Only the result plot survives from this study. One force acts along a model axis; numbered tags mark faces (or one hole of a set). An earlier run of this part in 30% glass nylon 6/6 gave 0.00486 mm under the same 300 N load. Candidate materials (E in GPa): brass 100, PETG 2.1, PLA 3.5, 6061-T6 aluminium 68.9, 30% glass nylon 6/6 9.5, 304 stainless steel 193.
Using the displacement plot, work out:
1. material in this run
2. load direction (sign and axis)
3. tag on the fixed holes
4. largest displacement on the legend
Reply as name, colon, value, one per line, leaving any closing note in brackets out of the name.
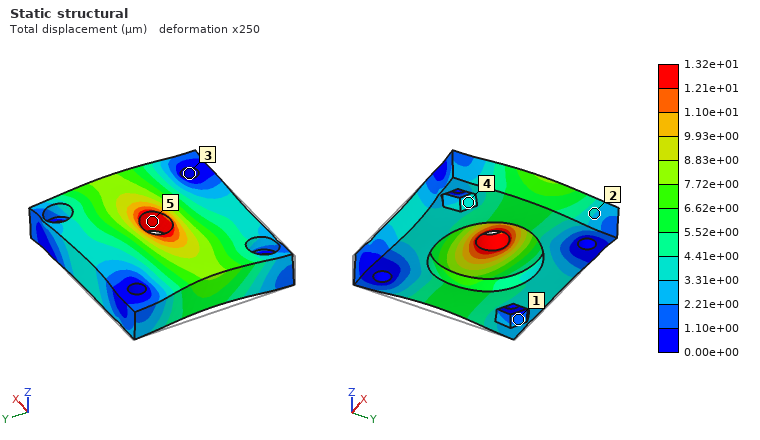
material in this run: PLA
load direction: +X
tag on the fixed holes: 3
largest displacement on the legend: 1.32e+01 µm
